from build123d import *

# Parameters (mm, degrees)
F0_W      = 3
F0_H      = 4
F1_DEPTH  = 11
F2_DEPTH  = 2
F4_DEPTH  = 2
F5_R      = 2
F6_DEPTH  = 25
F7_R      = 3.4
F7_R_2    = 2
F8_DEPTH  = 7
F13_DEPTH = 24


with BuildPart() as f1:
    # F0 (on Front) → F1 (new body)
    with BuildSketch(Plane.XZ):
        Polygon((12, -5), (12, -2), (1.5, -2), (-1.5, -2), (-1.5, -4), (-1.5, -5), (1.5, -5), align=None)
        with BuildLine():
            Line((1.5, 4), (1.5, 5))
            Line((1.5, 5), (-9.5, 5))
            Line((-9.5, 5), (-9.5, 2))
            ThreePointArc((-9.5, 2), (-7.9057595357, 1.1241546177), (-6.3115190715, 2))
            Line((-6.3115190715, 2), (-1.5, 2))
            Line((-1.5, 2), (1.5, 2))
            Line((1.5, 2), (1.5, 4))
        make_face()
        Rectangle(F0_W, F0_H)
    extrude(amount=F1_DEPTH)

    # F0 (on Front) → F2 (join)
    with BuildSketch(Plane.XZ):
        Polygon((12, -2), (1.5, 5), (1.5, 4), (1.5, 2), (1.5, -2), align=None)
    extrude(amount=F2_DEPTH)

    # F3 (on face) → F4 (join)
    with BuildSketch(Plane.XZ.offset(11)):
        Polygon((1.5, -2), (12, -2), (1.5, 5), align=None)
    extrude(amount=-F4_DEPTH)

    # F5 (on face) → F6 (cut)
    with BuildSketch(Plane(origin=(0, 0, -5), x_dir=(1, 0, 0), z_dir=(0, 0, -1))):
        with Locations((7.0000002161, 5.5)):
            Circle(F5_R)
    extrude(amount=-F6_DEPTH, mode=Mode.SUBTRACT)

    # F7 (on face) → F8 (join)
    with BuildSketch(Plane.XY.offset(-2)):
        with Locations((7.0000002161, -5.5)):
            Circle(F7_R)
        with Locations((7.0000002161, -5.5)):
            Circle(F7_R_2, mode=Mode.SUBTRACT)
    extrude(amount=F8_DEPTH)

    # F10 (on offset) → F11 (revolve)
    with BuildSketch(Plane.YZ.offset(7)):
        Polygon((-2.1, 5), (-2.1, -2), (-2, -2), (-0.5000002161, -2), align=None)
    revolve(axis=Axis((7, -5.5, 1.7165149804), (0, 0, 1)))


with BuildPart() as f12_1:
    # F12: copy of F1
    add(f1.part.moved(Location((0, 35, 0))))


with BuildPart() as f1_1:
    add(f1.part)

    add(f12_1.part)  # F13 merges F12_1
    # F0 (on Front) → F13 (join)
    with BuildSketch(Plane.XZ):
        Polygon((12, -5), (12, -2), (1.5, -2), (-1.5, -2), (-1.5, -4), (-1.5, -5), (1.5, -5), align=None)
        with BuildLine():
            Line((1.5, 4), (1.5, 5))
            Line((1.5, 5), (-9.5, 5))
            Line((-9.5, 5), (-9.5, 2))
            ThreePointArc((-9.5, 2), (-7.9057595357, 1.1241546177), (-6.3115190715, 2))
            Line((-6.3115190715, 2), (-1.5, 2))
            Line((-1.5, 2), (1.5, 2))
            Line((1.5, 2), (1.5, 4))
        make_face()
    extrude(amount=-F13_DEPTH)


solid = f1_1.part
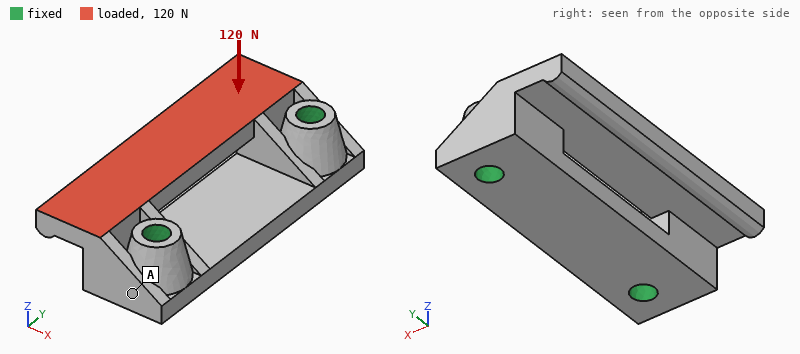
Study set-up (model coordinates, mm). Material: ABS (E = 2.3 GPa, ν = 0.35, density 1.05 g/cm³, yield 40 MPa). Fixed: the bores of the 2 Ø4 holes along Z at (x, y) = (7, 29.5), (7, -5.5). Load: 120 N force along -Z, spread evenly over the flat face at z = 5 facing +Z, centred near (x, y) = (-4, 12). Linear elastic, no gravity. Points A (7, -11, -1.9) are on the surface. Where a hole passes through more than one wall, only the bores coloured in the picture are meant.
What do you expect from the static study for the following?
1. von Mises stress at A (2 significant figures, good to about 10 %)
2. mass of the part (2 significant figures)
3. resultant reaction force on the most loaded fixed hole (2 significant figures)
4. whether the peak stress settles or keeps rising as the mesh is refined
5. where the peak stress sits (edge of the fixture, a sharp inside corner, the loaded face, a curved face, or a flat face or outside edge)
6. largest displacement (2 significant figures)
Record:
1.9 MPa
4.7 g
61 N
keeps rising
a sharp inside corner
0.32 mm
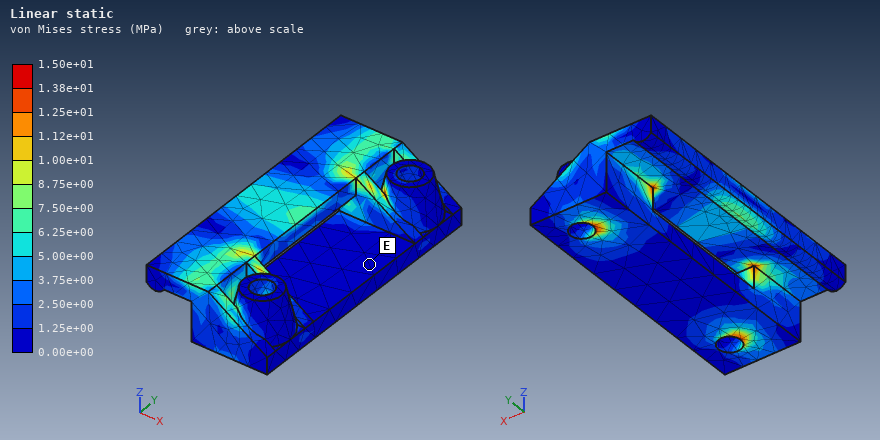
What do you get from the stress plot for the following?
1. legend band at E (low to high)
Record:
0.00e+00 to 1.25e+00 MPa
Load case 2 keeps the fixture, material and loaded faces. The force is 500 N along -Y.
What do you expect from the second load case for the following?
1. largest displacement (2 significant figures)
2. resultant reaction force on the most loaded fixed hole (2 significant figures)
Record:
0.24 mm
270 N
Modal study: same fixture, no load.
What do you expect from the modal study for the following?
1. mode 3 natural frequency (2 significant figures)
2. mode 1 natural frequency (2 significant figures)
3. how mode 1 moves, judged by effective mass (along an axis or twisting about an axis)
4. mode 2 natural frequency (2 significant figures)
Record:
5600 Hz
3000 Hz
along Z
5000 Hz
